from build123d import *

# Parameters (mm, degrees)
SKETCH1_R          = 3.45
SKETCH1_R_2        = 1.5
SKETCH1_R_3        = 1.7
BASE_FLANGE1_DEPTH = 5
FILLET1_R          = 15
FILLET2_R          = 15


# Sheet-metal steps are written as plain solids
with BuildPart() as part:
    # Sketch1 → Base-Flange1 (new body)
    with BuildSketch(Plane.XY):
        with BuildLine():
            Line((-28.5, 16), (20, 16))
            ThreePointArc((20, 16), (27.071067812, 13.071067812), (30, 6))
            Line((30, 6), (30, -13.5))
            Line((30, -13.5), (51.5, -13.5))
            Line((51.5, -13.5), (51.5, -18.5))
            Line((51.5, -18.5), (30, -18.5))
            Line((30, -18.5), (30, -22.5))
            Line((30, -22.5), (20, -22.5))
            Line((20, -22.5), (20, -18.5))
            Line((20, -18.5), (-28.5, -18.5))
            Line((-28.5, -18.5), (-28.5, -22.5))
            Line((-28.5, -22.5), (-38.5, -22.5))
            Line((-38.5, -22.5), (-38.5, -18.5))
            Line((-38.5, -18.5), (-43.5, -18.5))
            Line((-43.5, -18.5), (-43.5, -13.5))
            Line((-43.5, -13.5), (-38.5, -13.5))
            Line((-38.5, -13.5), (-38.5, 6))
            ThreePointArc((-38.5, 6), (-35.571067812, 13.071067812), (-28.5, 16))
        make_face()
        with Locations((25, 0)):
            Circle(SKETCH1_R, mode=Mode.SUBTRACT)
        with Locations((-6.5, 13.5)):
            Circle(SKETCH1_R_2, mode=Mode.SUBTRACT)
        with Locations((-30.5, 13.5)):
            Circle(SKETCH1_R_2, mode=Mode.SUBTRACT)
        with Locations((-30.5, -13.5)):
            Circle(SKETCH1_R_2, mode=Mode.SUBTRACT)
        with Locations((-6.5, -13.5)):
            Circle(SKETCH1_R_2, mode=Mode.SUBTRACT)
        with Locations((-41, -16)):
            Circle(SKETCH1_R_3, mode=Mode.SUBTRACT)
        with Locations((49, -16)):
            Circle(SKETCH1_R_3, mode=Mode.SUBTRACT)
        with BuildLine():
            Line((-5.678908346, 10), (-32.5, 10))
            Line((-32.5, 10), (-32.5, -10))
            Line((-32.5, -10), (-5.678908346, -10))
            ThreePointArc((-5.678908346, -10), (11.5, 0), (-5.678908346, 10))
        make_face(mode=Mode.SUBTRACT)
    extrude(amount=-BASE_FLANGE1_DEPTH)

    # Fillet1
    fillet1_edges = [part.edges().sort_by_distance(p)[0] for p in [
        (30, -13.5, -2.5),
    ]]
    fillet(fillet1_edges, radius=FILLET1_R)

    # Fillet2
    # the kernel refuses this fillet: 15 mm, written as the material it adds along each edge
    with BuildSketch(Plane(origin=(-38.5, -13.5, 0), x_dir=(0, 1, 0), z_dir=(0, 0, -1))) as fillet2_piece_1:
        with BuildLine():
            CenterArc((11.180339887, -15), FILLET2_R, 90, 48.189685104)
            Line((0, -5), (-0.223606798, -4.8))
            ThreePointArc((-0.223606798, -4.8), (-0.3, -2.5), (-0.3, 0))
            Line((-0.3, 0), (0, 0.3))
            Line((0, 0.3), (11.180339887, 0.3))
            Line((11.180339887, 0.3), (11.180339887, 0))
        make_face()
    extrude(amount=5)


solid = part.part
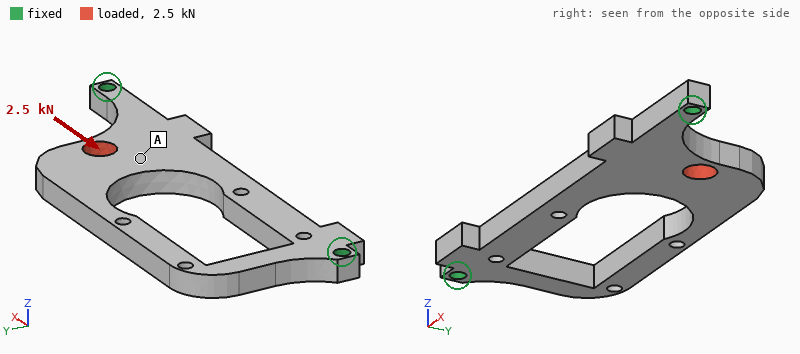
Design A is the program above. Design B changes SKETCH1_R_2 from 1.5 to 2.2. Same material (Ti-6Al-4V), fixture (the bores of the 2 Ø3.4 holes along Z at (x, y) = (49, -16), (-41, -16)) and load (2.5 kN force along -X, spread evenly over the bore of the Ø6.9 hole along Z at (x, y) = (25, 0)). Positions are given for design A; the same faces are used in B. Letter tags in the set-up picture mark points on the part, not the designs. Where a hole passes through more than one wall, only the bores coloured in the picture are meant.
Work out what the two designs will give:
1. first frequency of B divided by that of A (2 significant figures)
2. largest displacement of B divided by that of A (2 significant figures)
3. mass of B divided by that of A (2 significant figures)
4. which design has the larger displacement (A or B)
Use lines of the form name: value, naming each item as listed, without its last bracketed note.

first frequency of B divided by that of A: 0.98
largest displacement of B divided by that of A: 1.2
mass of B divided by that of A: 0.98
which design has the larger displacement: B
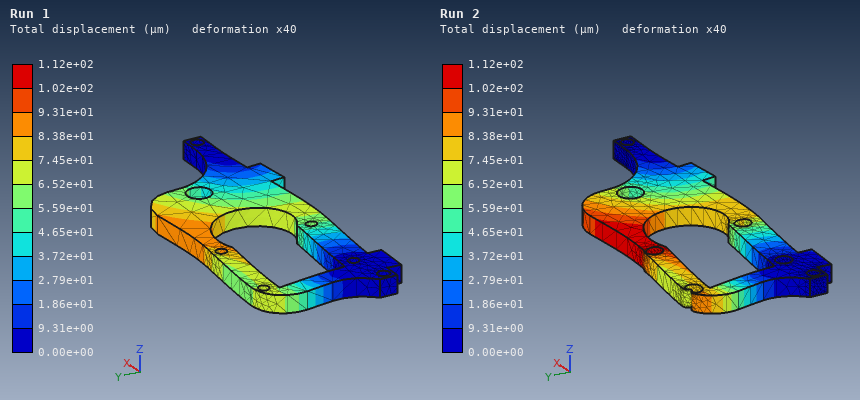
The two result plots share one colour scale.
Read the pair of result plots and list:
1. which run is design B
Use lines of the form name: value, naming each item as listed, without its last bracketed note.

which run is design B: Run 2
